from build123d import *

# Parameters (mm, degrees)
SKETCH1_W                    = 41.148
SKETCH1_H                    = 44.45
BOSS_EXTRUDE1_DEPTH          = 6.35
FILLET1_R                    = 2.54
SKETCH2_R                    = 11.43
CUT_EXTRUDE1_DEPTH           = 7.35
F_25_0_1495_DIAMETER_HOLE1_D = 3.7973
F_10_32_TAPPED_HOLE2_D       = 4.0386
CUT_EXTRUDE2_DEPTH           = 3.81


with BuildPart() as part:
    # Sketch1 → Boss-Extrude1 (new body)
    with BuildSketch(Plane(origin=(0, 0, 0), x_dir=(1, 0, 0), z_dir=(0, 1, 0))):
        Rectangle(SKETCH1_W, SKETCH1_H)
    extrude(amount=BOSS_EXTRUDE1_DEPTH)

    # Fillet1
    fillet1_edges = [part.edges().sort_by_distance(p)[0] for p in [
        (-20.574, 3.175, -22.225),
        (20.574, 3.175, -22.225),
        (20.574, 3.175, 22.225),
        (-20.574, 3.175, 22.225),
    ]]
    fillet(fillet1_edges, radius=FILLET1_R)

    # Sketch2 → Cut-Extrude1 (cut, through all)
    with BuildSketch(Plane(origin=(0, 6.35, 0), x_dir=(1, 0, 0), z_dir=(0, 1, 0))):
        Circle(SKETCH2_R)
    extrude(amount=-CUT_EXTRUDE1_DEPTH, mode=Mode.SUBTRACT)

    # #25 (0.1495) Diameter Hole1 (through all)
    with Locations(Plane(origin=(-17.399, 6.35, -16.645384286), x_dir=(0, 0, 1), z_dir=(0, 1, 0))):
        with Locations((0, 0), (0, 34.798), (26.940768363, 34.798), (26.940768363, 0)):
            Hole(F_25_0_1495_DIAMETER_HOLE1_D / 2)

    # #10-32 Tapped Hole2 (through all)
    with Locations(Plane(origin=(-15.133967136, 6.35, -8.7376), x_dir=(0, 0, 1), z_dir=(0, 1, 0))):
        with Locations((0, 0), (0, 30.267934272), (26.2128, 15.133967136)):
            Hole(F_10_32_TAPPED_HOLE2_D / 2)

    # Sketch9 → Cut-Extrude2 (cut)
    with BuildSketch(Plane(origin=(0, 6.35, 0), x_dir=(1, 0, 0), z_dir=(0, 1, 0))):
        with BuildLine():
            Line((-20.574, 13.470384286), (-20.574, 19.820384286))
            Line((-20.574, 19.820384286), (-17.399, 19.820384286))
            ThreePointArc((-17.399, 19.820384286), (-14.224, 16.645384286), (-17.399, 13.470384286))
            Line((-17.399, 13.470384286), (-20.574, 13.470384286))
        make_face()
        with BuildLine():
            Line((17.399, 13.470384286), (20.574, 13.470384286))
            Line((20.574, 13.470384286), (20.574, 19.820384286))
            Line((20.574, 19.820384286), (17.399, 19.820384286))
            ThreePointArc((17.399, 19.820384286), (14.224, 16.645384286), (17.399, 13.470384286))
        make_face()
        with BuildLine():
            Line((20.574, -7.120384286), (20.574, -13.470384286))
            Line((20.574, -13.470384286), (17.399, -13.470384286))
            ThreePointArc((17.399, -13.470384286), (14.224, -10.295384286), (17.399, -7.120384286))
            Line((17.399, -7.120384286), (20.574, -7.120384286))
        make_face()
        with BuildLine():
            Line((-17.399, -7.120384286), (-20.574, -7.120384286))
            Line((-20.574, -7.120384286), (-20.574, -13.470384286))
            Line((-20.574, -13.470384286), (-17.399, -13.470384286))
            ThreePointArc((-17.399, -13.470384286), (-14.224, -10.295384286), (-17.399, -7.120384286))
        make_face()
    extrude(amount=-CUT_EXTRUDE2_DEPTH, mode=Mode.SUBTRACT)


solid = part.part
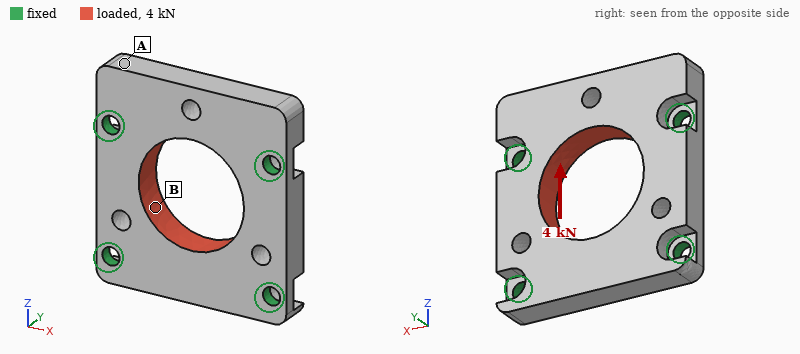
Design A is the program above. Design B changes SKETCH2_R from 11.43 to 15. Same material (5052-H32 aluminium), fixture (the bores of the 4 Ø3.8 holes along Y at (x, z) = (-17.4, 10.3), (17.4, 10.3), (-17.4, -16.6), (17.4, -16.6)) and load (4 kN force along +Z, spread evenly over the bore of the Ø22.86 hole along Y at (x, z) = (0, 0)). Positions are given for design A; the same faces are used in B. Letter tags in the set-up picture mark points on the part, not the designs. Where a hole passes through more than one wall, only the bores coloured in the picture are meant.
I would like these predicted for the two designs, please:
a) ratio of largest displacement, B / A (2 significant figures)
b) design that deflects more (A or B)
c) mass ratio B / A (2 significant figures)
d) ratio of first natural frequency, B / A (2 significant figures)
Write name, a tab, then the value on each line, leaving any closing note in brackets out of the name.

ratio of largest displacement, B / A	1.5
design that deflects more	B
mass ratio B / A	0.77
ratio of first natural frequency, B / A	0.87
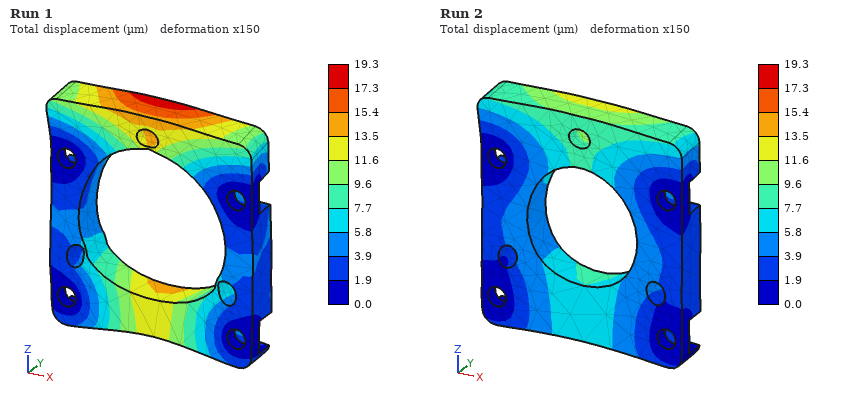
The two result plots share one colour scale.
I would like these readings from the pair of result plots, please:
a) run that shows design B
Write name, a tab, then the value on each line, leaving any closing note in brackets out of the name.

run that shows design B	Run 1
